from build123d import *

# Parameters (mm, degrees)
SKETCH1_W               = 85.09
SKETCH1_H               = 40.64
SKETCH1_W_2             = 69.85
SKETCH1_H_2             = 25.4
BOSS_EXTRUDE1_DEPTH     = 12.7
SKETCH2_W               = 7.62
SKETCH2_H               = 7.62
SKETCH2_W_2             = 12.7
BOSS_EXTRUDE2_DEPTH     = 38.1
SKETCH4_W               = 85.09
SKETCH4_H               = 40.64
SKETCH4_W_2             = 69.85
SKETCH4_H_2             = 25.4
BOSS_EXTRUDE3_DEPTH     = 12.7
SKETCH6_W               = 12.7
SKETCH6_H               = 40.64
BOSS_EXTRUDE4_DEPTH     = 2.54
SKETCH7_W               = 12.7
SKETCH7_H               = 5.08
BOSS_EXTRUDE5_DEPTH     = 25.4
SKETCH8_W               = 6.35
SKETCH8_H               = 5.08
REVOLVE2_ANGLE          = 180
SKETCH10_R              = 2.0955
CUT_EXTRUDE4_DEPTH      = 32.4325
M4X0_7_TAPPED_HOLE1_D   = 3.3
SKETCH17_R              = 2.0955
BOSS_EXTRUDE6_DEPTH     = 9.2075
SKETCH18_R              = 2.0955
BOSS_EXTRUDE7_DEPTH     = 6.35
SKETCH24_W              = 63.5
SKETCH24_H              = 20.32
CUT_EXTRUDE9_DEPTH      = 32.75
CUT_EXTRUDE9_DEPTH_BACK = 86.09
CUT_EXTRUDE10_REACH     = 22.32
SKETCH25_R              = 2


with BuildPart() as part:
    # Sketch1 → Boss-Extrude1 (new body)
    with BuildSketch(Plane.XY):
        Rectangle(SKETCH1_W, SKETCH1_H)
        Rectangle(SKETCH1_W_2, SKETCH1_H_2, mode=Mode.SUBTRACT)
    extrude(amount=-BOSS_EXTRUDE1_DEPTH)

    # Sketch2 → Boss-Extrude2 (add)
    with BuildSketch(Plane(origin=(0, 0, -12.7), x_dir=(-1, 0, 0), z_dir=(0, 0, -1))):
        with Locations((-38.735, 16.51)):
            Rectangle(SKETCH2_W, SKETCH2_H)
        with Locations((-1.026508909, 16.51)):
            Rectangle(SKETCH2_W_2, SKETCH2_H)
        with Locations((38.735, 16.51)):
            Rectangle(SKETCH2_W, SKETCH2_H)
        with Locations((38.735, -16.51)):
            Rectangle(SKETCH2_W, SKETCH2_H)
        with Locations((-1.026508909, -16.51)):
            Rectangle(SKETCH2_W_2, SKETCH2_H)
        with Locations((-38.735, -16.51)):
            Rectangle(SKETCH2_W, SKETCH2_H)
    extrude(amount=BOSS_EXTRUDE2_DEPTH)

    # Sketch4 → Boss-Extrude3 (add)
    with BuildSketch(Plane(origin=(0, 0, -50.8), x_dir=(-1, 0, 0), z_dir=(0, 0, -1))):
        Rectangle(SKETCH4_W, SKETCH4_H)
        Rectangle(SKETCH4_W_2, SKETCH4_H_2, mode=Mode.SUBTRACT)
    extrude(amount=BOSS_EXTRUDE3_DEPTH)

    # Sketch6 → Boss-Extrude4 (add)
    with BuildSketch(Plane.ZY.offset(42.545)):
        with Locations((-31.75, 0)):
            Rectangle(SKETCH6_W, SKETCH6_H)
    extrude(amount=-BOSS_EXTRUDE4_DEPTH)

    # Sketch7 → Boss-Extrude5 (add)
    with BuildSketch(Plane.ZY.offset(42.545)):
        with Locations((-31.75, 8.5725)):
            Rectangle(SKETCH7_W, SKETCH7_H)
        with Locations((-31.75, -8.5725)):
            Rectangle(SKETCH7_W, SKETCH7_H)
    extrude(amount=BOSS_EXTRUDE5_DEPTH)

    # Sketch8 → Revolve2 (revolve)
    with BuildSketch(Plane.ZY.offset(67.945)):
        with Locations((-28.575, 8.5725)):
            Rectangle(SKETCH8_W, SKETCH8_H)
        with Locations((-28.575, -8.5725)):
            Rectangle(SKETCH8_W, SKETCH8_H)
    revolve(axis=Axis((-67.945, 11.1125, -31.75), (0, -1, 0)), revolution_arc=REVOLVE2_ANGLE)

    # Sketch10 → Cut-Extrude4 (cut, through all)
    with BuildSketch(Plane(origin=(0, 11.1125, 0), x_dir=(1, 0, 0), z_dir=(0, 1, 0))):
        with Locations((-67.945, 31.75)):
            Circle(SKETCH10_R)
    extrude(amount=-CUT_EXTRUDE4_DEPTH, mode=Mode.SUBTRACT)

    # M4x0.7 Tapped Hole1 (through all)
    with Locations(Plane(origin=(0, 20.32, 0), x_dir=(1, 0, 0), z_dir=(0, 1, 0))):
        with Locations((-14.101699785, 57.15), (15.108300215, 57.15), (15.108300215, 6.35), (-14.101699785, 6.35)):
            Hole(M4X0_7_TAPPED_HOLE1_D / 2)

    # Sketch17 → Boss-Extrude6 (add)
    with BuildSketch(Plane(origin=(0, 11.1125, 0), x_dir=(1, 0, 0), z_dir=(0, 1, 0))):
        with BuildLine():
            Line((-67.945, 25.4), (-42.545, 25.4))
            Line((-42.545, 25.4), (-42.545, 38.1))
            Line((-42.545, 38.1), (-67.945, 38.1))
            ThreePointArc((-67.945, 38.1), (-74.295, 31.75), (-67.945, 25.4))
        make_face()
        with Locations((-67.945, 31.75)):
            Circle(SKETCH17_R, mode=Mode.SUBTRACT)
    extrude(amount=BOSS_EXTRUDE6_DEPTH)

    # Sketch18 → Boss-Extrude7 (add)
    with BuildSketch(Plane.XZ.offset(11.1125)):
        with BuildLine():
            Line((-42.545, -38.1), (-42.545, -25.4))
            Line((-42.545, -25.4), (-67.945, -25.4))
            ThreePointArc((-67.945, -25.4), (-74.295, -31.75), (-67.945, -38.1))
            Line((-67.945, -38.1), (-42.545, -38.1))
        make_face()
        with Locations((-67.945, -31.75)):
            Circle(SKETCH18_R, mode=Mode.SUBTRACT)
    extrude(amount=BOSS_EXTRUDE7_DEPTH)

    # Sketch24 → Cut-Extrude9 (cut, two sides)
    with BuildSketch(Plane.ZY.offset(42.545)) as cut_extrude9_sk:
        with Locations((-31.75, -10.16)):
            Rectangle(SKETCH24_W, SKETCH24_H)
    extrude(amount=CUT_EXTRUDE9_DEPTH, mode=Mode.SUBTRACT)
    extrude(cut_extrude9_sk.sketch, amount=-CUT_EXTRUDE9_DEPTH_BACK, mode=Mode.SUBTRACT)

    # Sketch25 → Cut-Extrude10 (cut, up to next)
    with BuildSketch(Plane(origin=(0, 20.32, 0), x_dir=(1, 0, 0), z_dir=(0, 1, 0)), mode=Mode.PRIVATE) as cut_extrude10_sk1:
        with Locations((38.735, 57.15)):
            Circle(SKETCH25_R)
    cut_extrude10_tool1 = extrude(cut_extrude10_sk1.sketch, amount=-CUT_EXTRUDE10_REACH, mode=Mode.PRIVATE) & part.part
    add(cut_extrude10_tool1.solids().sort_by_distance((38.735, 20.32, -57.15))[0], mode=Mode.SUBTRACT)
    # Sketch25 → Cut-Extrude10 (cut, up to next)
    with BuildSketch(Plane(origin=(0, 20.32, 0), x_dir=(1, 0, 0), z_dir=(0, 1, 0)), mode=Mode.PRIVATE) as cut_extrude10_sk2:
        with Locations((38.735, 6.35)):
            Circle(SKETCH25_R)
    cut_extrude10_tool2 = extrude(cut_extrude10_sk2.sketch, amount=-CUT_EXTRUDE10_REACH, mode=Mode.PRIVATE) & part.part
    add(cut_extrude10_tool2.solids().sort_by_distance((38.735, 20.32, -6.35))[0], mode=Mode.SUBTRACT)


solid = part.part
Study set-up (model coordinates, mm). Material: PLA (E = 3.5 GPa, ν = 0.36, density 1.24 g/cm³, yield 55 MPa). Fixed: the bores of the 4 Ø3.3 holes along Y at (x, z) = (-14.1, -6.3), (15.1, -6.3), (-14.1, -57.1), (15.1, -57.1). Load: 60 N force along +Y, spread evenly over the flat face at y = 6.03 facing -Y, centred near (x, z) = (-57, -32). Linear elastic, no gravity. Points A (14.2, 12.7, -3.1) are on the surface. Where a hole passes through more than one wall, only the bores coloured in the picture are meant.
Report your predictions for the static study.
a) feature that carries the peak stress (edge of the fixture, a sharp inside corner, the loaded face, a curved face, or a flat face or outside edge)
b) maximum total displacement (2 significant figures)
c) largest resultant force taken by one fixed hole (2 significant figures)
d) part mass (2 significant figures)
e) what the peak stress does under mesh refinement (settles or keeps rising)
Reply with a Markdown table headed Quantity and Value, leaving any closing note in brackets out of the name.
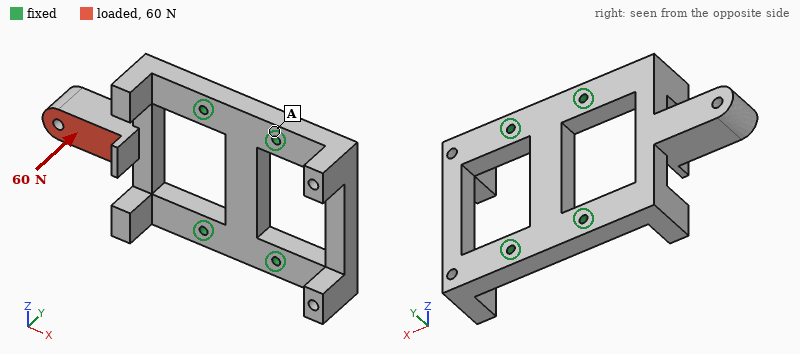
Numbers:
| Quantity | Value |
|---|---|
| feature that carries the peak stress | edge of the fixture |
| maximum total displacement | 1.4 mm |
| largest resultant force taken by one fixed hole | 38 N |
| part mass | 43 g |
| what the peak stress does under mesh refinement | keeps rising |
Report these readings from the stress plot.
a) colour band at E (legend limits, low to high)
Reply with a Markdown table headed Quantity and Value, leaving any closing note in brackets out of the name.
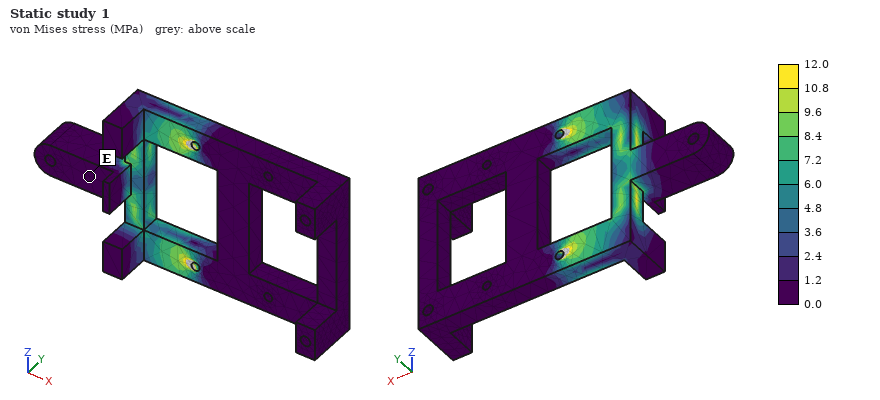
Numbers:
| Quantity | Value |
|---|---|
| colour band at E | 0.0 to 1.2 MPa |
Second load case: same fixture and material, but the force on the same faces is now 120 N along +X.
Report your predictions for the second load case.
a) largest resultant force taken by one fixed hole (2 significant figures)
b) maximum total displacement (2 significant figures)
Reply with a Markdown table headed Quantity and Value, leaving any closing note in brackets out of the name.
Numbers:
| Quantity | Value |
|---|---|
| largest resultant force taken by one fixed hole | 68 N |
| maximum total displacement | 1.2 mm |
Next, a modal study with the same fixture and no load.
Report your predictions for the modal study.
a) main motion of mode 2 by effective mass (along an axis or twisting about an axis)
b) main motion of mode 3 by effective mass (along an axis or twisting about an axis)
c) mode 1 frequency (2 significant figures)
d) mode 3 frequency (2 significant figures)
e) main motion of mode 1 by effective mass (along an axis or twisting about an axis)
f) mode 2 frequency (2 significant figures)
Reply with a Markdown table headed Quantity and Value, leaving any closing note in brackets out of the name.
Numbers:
| Quantity | Value |
|---|---|
| main motion of mode 2 by effective mass | along Y |
| main motion of mode 3 by effective mass | along Z |
| mode 1 frequency | 470 Hz |
| mode 3 frequency | 1500 Hz |
| main motion of mode 1 by effective mass | along Y |
| mode 2 frequency | 1300 Hz |
